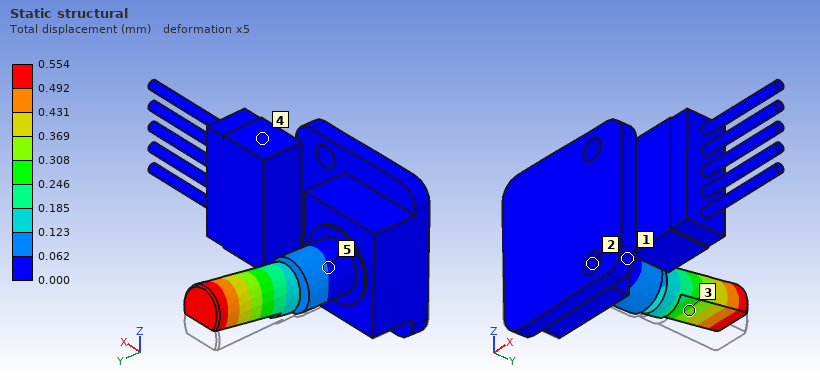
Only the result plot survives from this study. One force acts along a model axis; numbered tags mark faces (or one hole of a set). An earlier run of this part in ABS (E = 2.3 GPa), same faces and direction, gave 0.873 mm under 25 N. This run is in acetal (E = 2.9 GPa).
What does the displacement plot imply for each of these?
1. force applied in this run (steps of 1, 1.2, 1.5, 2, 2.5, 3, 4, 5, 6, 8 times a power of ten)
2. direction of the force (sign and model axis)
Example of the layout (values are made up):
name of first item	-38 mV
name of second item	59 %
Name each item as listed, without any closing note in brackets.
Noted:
force applied in this run	20 N
direction of the force	+Z
